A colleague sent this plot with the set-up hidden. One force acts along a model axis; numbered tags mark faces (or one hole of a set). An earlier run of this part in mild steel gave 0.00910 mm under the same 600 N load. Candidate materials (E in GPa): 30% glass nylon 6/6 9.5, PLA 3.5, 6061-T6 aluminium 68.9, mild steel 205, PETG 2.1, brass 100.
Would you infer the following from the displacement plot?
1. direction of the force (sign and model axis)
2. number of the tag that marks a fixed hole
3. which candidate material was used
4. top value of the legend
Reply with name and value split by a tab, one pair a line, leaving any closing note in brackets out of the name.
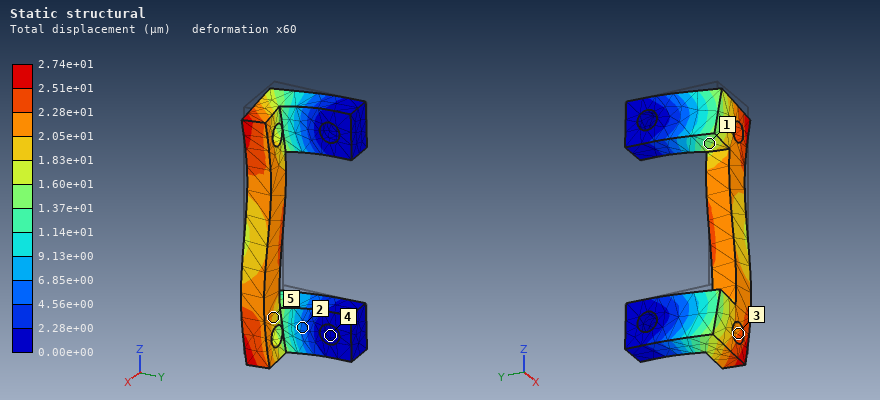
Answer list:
direction of the force	-Z
number of the tag that marks a fixed hole	4
which candidate material was used	6061-T6 aluminium
top value of the legend	2.74e+01 µm
